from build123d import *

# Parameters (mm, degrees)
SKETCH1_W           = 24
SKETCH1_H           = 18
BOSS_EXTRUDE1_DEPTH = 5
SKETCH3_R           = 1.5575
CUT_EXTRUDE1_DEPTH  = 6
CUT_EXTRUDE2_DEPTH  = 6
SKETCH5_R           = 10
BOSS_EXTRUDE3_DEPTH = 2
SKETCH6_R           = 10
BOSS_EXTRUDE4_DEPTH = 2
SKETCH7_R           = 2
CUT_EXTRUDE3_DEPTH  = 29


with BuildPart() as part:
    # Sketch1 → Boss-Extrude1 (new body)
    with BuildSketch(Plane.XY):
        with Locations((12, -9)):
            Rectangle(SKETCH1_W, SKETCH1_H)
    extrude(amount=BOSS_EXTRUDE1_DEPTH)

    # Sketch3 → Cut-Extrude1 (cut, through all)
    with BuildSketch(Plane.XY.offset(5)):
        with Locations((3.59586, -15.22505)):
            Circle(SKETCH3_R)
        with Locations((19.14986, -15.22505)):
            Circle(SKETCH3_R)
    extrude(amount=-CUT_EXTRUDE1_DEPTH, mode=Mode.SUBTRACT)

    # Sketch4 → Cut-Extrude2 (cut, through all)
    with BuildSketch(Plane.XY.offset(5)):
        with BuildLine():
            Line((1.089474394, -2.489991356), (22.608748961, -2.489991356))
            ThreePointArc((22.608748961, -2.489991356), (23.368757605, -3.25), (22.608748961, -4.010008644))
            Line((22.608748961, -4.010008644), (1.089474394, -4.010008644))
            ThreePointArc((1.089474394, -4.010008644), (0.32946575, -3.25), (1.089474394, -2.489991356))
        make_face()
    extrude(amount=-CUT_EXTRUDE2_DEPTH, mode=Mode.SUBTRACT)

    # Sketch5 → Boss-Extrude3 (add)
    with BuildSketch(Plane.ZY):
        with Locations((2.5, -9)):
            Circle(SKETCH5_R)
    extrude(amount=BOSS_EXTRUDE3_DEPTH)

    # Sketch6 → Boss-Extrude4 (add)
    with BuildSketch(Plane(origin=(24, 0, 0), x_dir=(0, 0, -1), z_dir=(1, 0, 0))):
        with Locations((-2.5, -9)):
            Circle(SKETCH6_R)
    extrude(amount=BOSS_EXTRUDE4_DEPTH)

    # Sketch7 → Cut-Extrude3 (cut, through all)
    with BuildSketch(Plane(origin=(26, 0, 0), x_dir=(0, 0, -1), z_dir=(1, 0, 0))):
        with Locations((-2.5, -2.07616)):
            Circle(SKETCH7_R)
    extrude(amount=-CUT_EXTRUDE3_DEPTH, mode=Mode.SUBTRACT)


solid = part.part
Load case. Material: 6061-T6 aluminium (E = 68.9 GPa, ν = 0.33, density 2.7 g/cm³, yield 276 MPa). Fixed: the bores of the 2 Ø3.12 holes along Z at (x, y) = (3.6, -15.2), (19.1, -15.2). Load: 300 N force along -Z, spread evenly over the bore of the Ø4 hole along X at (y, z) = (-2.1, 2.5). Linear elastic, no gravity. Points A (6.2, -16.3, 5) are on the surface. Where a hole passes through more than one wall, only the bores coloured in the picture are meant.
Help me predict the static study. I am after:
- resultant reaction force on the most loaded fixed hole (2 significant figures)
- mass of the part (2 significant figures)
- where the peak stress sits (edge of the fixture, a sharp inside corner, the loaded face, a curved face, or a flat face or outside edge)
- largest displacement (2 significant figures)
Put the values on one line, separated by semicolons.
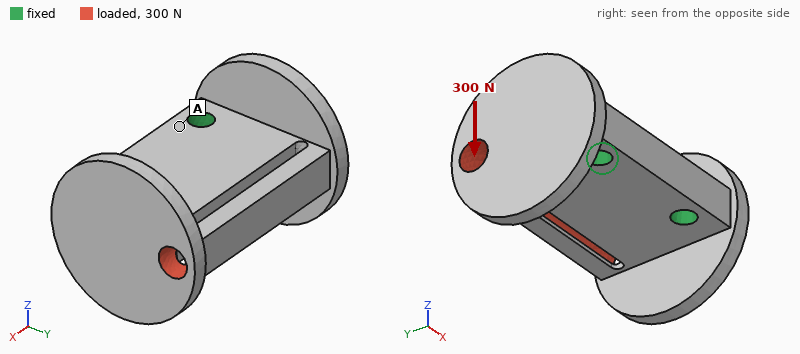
160 N; 7.9 g; the loaded face; 0.12 mm
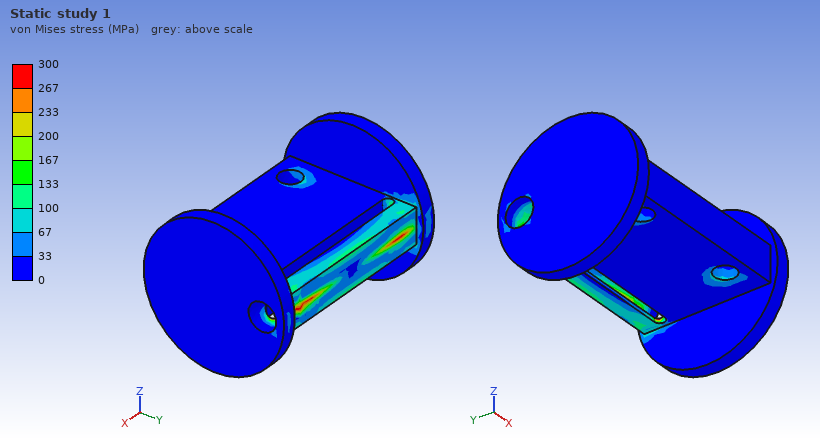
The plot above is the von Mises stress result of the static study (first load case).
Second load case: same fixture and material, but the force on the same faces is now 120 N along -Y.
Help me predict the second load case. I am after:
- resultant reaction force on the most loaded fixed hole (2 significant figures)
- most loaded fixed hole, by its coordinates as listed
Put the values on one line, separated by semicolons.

67 N; (19.1, -15.2)
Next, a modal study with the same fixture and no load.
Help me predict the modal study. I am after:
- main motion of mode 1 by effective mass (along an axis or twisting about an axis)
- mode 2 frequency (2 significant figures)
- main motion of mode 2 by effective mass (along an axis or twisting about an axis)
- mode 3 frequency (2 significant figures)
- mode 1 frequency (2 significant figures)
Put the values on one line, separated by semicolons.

along Z; 16 kHz; twisting about Y; 17 kHz; 14 kHz
